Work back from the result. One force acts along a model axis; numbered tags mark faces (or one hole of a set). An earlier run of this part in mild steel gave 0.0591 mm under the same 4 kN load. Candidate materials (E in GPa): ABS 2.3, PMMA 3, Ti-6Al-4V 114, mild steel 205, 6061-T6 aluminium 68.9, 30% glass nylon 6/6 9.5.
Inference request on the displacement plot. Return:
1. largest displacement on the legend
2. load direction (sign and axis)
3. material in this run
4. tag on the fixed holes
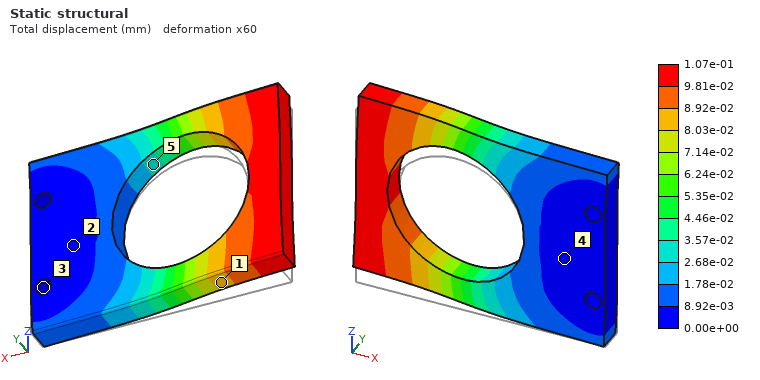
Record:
1.07e-01 mm
+Z
Ti-6Al-4V
3
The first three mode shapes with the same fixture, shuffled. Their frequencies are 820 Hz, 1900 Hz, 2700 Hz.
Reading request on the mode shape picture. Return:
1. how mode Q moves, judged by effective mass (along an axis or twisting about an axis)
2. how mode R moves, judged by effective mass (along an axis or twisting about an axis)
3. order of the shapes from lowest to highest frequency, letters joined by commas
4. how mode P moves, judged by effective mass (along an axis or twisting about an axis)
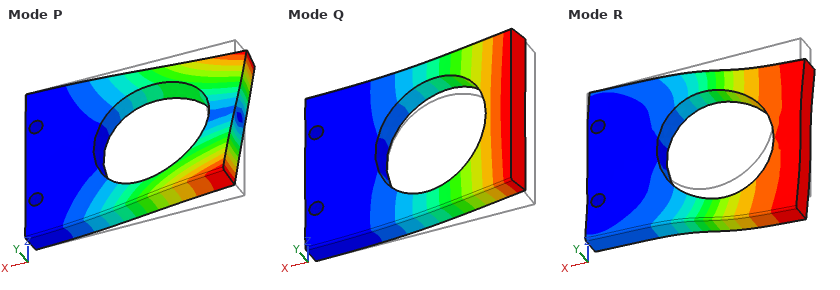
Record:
along Y
along Z
Q, P, R
twisting about X
